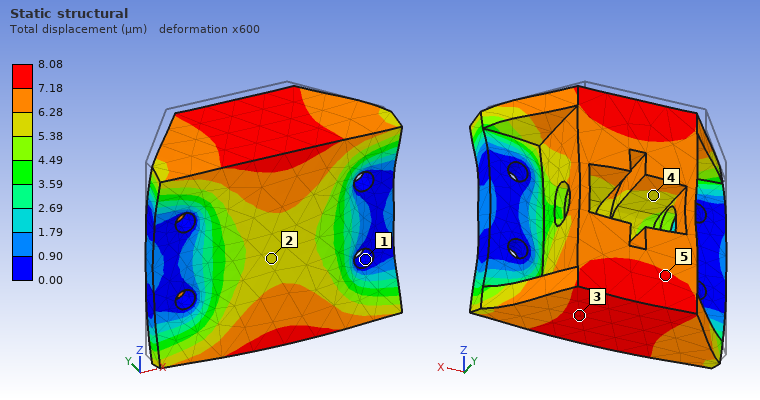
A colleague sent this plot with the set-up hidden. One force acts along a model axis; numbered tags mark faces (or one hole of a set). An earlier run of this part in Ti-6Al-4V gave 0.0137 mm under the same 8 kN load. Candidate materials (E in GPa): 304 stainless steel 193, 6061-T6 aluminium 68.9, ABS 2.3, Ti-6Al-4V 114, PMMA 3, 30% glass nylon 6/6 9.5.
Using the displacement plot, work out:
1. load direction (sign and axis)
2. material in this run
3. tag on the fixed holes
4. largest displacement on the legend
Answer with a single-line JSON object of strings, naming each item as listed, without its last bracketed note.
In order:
{"load direction": "-Y", "material in this run": "304 stainless steel", "tag on the fixed holes": "1", "largest displacement on the legend": "8.08 µm"}
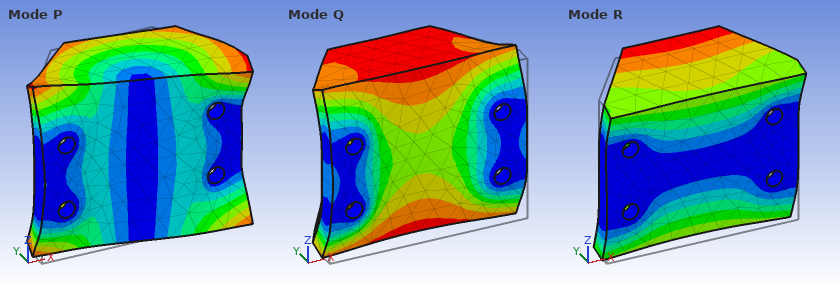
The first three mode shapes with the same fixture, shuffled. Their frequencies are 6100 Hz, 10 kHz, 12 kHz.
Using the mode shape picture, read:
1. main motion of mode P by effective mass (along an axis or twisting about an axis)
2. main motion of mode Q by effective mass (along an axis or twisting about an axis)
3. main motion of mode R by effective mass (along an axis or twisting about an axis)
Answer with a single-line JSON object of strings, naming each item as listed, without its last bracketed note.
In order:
{"main motion of mode P by effective mass": "along X", "main motion of mode Q by effective mass": "along Y", "main motion of mode R by effective mass": "along Z"}
